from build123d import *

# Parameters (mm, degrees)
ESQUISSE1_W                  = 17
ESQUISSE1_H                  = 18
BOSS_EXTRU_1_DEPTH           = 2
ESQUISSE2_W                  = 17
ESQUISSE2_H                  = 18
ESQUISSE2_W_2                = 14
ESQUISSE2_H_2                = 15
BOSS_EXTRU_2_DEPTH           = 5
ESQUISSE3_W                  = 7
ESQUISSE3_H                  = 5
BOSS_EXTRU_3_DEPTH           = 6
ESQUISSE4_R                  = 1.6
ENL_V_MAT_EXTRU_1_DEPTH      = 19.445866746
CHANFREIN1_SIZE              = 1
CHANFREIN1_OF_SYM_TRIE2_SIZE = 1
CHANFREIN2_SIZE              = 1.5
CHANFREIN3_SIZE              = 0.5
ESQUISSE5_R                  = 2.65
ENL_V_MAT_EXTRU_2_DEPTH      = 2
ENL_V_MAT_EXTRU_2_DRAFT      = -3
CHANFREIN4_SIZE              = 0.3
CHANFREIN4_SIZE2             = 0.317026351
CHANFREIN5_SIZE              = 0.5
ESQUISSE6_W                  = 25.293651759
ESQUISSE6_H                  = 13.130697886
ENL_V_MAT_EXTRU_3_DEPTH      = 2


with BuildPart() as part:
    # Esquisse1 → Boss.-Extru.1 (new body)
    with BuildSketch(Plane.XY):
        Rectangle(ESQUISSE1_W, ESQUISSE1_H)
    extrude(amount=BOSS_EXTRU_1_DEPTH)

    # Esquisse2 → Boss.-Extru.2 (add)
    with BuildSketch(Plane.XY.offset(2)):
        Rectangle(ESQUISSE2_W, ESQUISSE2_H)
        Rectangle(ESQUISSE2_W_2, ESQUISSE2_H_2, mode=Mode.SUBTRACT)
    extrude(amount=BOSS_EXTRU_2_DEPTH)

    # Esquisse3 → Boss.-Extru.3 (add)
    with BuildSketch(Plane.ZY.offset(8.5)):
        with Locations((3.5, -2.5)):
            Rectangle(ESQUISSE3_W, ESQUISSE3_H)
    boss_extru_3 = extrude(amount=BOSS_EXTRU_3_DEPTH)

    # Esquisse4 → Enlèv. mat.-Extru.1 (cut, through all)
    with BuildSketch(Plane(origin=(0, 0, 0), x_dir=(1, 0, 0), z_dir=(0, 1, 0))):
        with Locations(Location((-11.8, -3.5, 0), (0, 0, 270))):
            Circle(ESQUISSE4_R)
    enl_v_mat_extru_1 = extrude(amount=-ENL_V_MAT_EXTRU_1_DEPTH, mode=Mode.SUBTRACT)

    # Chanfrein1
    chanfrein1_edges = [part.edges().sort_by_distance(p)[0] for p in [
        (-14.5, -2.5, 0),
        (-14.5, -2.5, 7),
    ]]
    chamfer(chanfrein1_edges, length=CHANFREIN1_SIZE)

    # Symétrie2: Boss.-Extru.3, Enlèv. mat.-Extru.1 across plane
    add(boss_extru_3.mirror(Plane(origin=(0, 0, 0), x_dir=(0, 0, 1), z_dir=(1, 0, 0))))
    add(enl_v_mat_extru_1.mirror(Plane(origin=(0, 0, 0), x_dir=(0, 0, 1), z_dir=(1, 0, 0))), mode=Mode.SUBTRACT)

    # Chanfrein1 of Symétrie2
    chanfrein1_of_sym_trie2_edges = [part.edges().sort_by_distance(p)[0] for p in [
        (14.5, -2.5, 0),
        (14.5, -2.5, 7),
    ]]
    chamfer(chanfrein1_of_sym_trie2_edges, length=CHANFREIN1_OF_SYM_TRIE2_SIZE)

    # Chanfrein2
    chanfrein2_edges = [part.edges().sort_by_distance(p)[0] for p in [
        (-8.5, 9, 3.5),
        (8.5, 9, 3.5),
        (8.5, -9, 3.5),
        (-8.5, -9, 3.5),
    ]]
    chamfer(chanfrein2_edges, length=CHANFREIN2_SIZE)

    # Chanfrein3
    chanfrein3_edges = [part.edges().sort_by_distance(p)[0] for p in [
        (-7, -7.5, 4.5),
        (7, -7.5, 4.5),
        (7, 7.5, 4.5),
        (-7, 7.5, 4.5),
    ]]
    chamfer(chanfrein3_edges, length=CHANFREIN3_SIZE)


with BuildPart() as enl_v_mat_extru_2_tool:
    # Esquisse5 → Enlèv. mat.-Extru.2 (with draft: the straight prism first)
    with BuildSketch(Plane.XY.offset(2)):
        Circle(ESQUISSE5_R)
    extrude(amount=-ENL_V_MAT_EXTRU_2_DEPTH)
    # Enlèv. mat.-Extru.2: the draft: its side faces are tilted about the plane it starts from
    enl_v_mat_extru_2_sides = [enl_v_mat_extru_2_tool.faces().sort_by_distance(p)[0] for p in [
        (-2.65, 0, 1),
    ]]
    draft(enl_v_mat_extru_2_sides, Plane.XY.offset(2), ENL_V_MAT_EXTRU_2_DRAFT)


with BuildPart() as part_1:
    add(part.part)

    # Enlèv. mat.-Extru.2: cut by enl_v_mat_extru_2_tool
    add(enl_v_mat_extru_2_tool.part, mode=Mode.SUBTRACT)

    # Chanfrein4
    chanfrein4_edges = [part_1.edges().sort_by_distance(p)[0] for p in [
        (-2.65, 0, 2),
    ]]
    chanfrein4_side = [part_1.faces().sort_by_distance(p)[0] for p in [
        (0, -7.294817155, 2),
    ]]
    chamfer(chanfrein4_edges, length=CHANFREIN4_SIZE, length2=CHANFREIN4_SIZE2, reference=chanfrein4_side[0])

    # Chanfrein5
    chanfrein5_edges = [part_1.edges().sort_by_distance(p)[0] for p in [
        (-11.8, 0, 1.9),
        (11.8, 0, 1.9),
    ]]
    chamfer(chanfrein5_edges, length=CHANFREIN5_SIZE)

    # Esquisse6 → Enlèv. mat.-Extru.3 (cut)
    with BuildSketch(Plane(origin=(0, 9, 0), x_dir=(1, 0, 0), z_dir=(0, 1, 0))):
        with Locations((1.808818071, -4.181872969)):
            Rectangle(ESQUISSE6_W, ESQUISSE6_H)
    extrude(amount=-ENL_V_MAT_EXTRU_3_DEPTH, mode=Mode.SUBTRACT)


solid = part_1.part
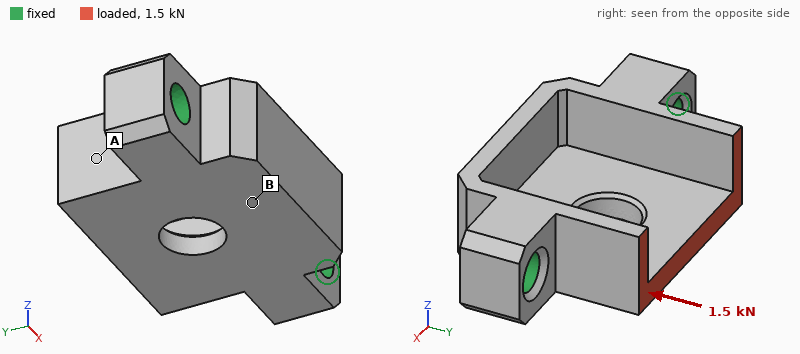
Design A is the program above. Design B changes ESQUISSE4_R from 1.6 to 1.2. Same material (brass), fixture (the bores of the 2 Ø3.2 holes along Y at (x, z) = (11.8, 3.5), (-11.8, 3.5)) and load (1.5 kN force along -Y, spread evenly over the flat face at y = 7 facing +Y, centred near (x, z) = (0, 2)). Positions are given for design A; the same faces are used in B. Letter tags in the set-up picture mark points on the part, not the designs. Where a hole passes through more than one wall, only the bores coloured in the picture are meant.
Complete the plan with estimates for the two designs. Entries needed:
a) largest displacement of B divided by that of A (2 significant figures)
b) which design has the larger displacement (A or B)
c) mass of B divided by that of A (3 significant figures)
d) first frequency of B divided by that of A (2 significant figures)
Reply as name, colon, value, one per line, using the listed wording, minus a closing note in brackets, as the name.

largest displacement of B divided by that of A: 1.1
which design has the larger displacement: B
mass of B divided by that of A: 1.03
first frequency of B divided by that of A: 0.96
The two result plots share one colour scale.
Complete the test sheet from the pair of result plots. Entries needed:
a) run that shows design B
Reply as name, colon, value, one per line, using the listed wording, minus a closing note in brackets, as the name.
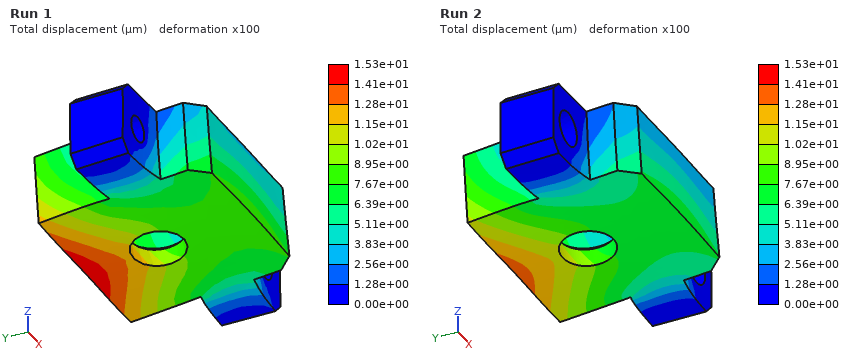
run that shows design B: Run 1
